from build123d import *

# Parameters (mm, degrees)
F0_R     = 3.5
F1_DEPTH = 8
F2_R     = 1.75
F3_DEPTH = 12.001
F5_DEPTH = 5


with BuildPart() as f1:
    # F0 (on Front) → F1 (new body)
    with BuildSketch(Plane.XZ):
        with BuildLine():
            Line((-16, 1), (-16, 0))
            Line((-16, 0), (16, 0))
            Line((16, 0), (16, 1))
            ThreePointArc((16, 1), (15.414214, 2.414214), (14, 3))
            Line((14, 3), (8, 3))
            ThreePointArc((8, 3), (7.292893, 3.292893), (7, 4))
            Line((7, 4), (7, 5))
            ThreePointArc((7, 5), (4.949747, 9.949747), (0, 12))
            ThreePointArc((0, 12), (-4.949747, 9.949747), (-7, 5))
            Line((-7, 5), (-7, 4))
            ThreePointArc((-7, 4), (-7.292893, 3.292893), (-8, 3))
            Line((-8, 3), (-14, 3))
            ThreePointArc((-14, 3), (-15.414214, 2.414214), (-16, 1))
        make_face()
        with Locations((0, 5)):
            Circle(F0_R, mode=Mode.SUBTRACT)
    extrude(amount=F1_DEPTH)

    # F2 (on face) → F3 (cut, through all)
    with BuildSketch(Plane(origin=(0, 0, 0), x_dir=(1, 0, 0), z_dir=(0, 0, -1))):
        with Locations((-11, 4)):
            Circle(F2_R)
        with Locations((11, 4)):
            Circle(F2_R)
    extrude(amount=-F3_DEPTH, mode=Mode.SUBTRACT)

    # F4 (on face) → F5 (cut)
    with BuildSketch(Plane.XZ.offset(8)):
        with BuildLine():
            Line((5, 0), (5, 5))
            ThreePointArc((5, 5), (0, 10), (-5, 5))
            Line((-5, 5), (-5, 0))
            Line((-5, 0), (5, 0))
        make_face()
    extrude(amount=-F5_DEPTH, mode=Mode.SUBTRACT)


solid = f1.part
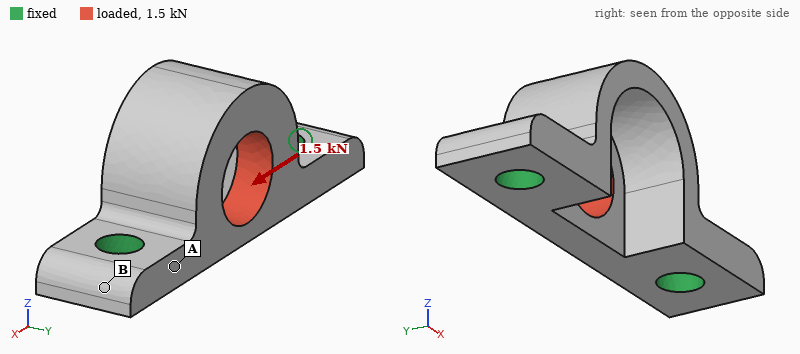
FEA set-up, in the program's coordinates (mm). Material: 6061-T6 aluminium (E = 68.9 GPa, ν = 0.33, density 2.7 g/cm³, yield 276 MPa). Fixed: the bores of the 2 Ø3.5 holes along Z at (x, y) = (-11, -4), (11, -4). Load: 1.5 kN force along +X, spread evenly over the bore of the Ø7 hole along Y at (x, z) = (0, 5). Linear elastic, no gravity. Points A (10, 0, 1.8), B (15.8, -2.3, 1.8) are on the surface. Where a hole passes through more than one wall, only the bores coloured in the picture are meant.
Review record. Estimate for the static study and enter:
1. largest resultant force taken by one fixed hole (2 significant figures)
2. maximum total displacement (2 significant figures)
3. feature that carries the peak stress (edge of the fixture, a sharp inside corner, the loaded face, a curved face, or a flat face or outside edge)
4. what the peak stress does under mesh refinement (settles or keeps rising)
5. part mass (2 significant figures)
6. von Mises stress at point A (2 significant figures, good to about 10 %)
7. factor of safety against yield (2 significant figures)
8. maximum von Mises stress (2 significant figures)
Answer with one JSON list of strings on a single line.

["800 N", "21 µm", "a curved face", "settles", "2.6 g", "39 MPa", "1.4", "190 MPa"]
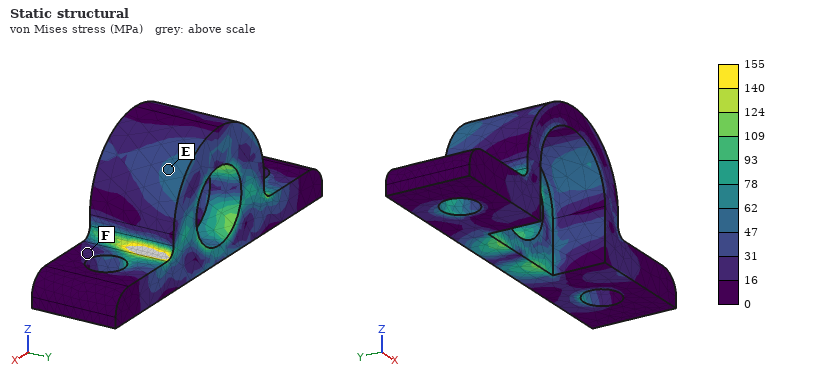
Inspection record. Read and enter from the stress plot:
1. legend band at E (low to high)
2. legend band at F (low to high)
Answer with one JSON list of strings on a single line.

["47 to 62 MPa", "16 to 31 MPa"]
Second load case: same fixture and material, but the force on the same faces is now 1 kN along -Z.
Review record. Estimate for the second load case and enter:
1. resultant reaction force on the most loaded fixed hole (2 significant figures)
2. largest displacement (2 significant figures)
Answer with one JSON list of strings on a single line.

["510 N", "35 µm"]
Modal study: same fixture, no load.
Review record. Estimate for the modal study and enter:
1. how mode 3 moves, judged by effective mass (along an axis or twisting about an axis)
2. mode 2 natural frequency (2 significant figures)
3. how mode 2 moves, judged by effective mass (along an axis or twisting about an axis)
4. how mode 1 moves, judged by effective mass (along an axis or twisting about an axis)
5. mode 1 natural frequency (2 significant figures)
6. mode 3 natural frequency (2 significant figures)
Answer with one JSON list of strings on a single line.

["along Z", "31 kHz", "along X", "along Y", "18 kHz", "41 kHz"]
